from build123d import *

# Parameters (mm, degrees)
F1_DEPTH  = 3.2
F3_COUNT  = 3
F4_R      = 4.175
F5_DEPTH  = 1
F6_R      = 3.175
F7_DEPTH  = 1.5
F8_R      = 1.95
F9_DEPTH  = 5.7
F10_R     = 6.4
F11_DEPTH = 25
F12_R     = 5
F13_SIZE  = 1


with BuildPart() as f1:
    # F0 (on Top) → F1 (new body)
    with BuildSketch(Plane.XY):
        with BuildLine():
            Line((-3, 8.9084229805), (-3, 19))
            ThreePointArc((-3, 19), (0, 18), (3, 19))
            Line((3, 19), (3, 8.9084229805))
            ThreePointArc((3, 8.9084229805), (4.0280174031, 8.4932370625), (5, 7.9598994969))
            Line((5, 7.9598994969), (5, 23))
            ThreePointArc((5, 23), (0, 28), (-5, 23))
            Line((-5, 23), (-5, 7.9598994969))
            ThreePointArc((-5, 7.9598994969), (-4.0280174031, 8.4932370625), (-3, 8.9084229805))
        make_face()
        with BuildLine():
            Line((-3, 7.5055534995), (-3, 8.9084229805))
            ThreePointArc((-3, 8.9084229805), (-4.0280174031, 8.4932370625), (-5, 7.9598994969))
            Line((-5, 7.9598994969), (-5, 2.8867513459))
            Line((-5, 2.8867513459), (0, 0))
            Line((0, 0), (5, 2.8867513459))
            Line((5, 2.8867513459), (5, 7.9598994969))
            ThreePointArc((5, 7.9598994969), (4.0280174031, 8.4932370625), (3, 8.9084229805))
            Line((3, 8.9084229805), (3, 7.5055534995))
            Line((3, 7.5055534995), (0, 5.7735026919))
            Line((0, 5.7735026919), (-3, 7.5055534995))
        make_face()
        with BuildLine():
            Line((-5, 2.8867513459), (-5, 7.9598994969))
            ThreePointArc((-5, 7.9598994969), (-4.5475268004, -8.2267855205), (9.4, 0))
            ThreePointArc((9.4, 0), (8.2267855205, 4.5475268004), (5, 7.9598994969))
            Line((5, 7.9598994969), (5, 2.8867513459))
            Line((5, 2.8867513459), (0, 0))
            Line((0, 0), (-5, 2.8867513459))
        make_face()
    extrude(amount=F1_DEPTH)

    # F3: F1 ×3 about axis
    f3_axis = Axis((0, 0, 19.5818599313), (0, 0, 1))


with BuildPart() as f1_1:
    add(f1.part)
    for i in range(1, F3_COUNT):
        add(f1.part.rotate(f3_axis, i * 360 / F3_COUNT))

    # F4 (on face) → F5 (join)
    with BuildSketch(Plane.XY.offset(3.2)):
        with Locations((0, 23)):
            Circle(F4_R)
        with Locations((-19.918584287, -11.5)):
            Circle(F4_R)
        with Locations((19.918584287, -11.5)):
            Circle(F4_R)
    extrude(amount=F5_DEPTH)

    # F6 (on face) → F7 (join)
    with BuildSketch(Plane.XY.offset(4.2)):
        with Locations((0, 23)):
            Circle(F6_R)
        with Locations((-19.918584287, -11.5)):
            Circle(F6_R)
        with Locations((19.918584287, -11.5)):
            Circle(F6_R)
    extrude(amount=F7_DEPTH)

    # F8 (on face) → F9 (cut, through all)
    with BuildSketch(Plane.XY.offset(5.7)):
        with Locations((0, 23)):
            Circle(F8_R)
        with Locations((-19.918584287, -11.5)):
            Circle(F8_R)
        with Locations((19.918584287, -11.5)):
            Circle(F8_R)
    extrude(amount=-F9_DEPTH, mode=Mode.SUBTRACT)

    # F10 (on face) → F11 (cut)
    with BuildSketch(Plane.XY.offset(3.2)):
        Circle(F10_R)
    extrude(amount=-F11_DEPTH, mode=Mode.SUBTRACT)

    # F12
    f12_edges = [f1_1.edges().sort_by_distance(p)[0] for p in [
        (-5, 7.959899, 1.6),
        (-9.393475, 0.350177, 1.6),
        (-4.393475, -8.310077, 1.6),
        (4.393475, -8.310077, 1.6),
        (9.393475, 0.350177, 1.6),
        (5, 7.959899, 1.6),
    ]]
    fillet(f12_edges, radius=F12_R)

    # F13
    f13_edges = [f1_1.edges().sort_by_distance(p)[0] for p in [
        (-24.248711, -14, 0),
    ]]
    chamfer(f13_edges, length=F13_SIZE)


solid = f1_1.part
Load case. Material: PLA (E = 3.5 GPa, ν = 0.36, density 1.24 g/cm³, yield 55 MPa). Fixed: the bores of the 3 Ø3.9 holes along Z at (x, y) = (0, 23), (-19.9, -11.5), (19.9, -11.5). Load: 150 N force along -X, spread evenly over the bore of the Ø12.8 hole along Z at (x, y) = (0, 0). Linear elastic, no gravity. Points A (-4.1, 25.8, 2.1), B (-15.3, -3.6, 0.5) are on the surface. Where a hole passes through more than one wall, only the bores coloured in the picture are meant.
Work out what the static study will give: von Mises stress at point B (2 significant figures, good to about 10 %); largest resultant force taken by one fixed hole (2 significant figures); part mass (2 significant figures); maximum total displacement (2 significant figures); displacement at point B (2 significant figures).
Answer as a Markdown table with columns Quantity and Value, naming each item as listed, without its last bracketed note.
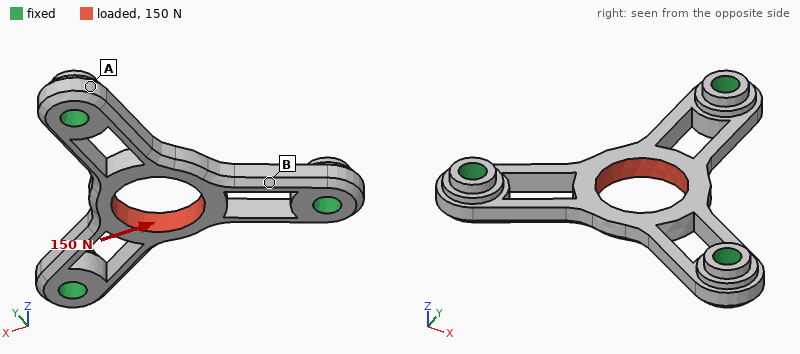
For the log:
| Quantity | Value |
|---|---|
| von Mises stress at point B | 9.1 MPa |
| largest resultant force taken by one fixed hole | 83 N |
| part mass | 2.1 g |
| maximum total displacement | 91 µm |
| displacement at point B | 25 µm |
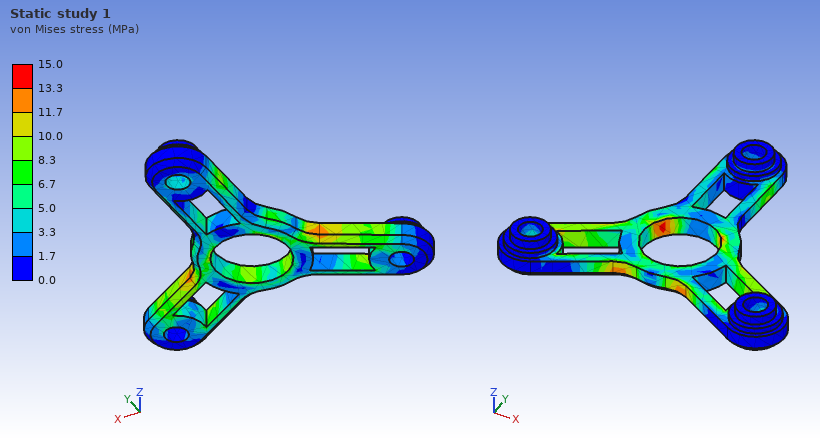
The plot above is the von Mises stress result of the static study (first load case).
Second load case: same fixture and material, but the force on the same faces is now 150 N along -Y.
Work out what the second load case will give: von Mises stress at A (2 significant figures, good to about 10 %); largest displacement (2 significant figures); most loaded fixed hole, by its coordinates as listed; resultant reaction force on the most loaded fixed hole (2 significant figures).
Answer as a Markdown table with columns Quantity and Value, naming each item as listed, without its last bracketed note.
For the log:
| Quantity | Value |
|---|---|
| von Mises stress at A | 1.2 MPa |
| largest displacement | 99 µm |
| most loaded fixed hole, by its coordinates as listed | (0, 23) |
| resultant reaction force on the most loaded fixed hole | 96 N |
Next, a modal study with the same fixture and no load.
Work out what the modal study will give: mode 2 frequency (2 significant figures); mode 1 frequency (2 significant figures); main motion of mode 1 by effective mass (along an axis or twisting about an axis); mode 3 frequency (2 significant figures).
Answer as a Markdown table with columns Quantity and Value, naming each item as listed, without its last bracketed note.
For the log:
| Quantity | Value |
|---|---|
| mode 2 frequency | 5200 Hz |
| mode 1 frequency | 3000 Hz |
| main motion of mode 1 by effective mass | along Z |
| mode 3 frequency | 5200 Hz |
